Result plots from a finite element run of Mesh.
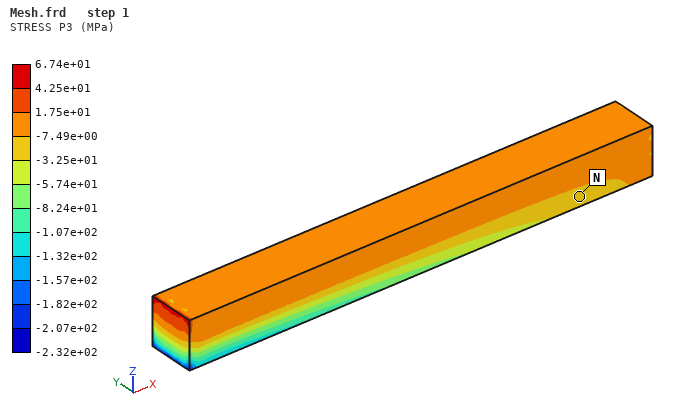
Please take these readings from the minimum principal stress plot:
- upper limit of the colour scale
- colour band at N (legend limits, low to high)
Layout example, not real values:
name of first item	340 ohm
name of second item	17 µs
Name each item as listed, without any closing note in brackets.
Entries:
upper limit of the colour scale	6.74e+01 MPa
colour band at N	-3.25e+01 to -7.49e+00 MPa
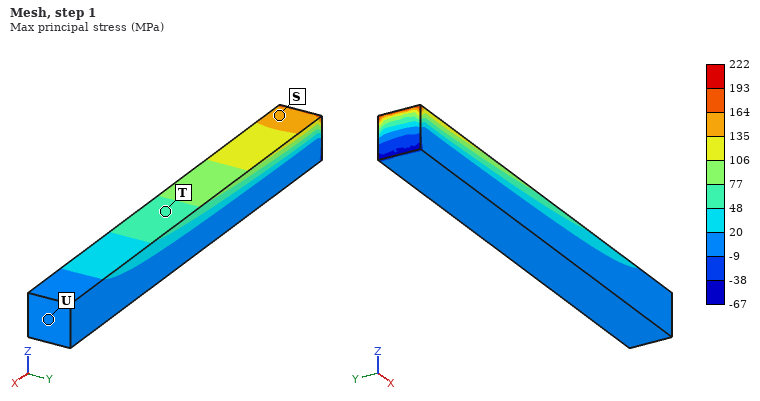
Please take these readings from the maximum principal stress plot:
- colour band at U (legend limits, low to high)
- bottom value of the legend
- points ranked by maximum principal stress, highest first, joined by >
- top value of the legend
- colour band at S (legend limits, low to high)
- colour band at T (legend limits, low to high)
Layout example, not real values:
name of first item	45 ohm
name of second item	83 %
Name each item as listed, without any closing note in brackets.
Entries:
colour band at U	-9 to 20 MPa
bottom value of the legend	-67 MPa
points ranked by maximum principal stress, highest first, joined by >	S > T > U
top value of the legend	222 MPa
colour band at S	135 to 164 MPa
colour band at T	48 to 77 MPa
